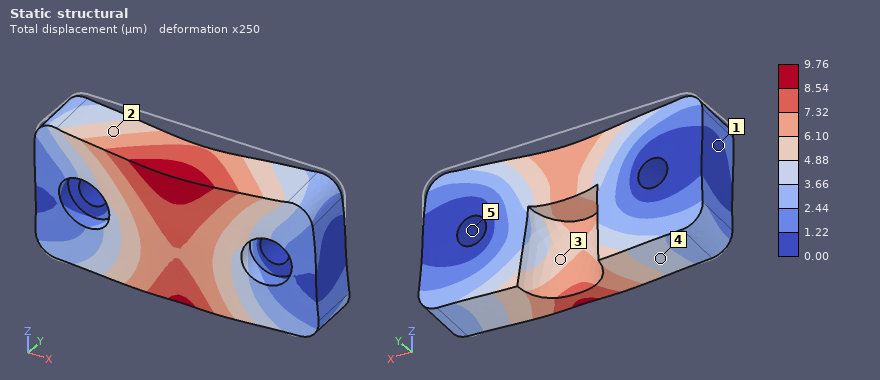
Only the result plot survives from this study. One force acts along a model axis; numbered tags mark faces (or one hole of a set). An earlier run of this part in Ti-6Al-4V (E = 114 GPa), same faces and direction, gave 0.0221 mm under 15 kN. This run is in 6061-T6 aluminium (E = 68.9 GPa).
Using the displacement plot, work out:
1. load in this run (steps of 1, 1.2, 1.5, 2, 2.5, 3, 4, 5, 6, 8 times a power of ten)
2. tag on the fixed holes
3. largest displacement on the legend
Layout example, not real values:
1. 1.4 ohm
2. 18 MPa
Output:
1. 4 kN
2. 5
3. 9.76 µm
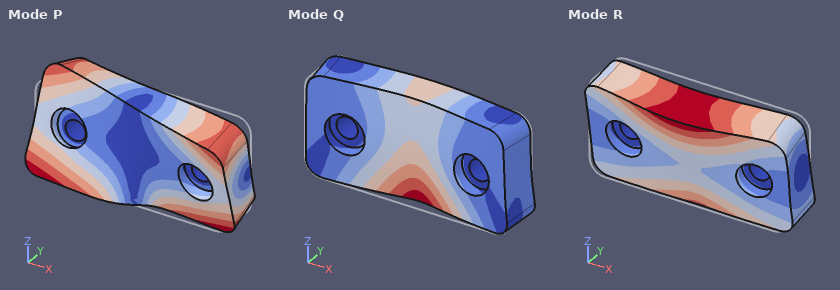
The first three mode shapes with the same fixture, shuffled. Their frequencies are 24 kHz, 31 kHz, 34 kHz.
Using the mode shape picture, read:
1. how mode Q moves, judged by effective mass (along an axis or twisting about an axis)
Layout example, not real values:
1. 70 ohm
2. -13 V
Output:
1. along Y
